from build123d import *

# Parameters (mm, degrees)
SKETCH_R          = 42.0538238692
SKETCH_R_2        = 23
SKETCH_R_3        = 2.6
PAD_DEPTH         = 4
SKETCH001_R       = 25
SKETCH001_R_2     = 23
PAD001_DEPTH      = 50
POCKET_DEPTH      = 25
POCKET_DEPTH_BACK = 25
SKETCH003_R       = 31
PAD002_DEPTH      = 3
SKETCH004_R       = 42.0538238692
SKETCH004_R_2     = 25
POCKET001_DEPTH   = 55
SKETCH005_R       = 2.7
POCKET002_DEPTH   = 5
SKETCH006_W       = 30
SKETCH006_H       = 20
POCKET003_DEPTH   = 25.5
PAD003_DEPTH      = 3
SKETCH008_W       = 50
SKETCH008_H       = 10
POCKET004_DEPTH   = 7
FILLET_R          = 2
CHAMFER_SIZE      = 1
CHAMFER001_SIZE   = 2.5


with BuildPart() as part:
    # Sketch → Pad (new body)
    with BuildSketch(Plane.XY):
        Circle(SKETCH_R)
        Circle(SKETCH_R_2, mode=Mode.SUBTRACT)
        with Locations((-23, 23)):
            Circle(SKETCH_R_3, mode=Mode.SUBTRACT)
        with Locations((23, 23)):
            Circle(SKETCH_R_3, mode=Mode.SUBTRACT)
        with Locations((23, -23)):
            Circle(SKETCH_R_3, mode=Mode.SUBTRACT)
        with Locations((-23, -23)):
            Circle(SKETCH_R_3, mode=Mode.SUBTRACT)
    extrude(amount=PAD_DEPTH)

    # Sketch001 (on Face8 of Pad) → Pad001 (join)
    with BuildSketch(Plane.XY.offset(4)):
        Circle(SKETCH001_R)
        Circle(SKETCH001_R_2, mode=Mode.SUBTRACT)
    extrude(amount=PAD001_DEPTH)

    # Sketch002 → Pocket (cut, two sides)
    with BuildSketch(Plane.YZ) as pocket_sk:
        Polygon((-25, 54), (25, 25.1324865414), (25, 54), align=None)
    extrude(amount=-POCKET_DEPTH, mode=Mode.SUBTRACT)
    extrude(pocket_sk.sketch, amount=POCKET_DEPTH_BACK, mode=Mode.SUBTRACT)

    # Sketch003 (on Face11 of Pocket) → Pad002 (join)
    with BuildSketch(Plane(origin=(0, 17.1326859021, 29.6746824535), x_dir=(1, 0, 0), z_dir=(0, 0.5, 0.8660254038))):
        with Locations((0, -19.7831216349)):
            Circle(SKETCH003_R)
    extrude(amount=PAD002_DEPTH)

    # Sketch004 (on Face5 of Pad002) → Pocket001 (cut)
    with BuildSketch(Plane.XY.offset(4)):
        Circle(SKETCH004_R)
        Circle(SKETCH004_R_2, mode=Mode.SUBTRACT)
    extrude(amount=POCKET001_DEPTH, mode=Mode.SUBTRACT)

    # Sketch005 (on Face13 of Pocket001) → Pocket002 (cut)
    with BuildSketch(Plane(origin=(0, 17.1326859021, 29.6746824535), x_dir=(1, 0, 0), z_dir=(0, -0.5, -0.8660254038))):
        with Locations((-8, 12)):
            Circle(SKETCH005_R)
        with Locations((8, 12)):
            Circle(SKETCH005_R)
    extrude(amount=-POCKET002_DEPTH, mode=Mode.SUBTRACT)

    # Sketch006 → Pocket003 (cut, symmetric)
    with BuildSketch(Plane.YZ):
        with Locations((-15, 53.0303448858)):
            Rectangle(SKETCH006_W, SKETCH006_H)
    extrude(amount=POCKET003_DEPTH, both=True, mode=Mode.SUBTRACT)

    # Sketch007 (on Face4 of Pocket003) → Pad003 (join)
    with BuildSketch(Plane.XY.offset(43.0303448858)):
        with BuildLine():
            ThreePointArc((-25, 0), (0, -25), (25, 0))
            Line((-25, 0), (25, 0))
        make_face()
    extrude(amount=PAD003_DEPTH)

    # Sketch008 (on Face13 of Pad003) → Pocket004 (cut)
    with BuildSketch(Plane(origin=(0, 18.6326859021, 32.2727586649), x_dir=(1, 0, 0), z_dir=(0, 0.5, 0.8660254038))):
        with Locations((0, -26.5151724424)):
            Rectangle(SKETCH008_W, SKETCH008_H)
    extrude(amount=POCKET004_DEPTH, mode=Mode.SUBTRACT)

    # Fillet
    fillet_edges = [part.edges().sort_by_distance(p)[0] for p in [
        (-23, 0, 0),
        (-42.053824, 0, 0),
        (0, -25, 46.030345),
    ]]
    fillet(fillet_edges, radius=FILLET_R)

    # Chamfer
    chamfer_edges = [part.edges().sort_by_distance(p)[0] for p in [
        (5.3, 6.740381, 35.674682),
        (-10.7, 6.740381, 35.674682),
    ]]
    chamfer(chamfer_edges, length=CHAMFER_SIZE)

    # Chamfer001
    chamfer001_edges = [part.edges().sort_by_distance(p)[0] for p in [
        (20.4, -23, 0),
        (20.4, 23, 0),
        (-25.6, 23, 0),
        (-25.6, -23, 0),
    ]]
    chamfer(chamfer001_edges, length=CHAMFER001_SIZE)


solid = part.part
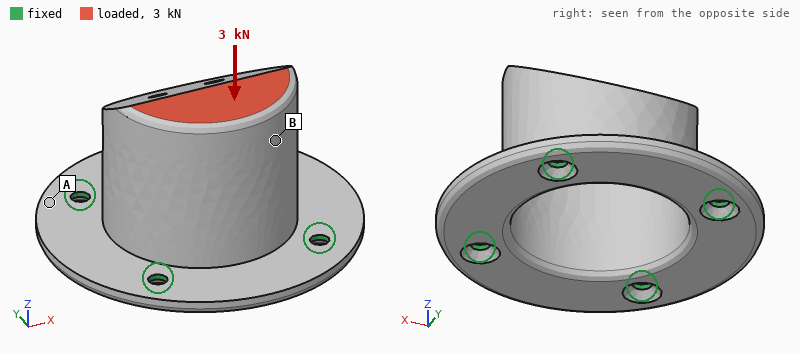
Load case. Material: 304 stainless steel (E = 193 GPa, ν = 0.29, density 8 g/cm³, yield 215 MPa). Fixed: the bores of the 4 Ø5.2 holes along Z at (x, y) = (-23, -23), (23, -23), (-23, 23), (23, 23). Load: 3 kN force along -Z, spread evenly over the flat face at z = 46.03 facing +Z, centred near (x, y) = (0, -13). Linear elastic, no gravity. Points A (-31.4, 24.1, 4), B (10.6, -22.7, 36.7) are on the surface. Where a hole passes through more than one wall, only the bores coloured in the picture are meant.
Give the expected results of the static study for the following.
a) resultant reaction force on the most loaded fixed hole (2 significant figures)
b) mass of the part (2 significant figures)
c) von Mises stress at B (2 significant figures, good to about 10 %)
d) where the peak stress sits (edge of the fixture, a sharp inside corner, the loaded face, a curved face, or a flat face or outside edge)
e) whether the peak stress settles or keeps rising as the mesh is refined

1.2 kN
250 g
33 MPa
edge of the fixture
keeps rising
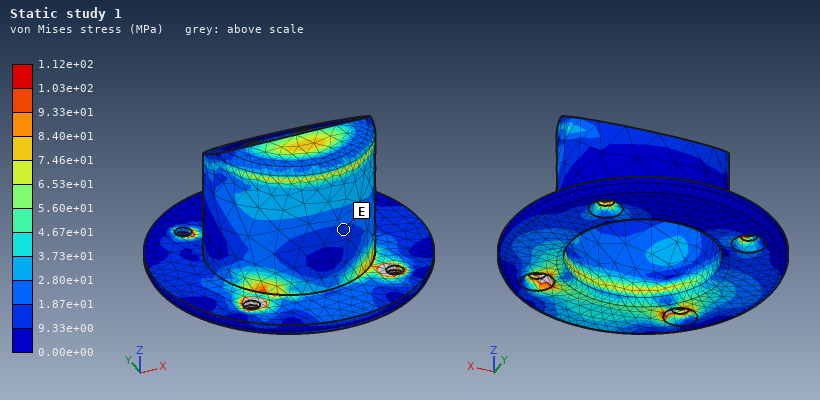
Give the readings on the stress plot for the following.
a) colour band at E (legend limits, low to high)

9.33e+00 to 1.87e+01 MPa
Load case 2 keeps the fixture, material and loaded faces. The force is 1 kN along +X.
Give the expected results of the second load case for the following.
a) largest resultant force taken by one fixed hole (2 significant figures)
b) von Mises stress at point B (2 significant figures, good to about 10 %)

650 N
12 MPa
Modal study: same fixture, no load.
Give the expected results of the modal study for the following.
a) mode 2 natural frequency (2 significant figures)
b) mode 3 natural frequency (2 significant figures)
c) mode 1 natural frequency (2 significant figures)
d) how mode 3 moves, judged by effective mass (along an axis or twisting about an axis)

4000 Hz
6200 Hz
4000 Hz
along Z
